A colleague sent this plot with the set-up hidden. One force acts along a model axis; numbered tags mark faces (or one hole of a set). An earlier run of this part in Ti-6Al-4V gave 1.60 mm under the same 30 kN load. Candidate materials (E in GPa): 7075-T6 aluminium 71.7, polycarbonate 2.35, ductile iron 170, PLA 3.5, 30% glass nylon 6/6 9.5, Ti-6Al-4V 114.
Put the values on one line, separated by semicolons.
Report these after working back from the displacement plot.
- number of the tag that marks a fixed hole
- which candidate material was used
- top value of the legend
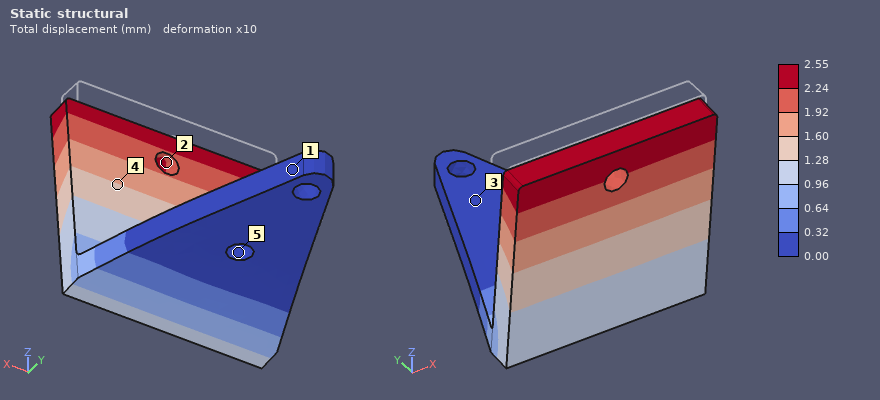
5; 7075-T6 aluminium; 2.55 mm
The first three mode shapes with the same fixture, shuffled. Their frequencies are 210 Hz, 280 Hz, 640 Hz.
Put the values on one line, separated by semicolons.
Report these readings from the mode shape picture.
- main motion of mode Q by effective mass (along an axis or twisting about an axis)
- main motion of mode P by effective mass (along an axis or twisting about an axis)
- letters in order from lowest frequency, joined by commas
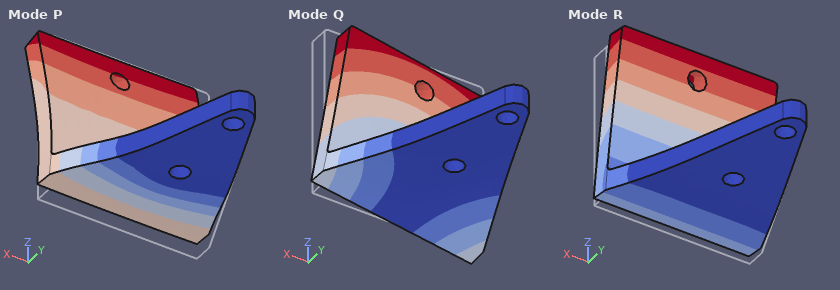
along X; along Z; R, Q, P
